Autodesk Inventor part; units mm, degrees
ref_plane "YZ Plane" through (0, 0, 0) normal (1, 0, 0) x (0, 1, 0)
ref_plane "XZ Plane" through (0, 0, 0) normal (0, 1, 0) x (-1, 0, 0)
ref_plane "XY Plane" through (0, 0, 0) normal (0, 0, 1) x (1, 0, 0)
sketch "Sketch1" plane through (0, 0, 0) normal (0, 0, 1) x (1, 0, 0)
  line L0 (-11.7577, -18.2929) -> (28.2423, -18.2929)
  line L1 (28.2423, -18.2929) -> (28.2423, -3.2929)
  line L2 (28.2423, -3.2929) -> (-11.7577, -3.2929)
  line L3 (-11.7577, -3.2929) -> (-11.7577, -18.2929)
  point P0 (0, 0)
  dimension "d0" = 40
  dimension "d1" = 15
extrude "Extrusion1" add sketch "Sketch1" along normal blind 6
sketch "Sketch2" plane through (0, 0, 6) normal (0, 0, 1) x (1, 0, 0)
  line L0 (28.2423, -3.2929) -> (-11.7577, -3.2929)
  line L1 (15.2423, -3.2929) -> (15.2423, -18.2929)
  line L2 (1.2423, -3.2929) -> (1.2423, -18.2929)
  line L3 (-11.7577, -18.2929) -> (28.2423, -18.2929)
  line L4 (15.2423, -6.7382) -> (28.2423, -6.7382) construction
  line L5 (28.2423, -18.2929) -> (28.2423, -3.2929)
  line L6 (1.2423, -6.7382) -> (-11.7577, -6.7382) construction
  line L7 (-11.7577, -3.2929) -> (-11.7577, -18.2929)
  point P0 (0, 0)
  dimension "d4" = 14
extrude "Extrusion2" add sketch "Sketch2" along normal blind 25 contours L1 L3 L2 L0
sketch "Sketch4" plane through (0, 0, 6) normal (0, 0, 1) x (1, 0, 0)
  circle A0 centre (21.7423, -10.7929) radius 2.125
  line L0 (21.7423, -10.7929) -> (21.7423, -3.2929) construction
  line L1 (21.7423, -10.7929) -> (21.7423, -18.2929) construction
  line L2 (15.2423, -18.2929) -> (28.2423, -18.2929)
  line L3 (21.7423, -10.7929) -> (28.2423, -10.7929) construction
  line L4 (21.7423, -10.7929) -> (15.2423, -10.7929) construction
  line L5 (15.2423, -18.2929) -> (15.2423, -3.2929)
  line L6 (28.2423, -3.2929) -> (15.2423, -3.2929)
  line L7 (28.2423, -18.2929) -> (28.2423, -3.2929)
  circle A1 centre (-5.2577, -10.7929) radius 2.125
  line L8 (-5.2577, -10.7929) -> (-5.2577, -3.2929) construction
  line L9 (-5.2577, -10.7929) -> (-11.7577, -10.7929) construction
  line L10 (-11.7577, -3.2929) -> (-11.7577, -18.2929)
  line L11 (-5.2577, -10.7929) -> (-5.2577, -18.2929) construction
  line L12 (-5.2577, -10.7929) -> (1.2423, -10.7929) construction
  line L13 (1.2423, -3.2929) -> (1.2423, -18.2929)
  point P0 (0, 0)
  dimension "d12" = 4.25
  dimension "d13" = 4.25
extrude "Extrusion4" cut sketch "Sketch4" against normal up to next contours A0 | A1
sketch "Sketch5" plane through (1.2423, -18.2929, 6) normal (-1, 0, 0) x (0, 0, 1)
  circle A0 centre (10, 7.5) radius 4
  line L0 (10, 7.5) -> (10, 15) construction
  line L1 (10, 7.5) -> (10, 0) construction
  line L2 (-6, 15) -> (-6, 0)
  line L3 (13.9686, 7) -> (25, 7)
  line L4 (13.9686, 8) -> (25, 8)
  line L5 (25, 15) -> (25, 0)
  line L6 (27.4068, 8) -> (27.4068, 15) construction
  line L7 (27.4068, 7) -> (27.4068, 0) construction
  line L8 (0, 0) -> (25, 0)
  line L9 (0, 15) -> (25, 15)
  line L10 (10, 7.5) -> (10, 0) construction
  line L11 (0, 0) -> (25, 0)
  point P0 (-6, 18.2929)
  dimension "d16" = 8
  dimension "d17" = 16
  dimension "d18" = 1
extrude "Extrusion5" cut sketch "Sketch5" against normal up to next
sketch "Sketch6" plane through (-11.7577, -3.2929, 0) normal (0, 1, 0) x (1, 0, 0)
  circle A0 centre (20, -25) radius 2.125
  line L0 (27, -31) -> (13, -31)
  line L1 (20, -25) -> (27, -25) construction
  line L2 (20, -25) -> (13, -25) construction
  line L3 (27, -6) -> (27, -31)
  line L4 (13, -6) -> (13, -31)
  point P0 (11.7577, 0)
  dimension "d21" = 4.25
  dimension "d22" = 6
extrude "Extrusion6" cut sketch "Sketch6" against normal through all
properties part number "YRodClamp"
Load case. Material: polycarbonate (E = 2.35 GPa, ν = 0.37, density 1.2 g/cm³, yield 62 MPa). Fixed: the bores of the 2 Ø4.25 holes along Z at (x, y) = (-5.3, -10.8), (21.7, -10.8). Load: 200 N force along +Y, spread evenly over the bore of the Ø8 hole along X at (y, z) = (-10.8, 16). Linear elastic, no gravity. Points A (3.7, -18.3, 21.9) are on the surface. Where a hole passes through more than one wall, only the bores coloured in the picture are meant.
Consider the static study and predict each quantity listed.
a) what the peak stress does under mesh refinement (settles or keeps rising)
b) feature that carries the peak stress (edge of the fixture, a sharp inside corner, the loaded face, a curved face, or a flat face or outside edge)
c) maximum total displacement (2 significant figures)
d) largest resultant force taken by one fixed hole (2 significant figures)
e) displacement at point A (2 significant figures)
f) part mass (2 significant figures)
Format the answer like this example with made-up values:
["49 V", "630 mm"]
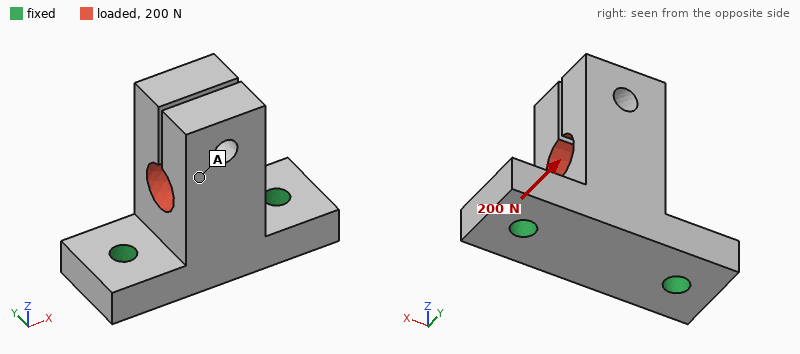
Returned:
["keeps rising", "edge of the fixture", "0.54 mm", "100 N", "0.35 mm", "9.1 g"]
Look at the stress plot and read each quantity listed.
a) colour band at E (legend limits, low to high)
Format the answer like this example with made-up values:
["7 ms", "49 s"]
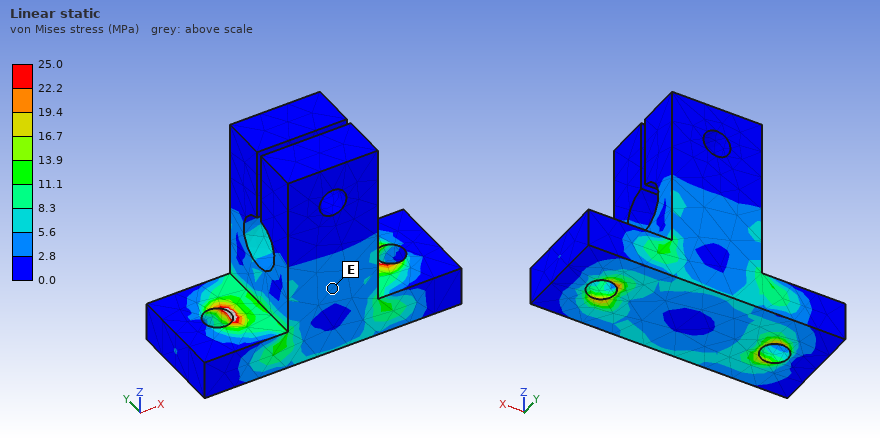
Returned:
["2.8 to 5.6 MPa"]
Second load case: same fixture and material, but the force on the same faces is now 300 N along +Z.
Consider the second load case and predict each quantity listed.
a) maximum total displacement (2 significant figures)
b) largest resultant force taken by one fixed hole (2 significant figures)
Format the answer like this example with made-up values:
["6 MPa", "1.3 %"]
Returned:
["0.19 mm", "160 N"]
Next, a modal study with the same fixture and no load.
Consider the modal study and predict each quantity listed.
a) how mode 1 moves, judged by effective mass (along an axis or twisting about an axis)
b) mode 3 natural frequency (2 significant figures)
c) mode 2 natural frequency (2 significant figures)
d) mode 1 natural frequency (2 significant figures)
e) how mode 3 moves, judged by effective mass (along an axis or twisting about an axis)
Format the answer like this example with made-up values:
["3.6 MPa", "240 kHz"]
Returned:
["along Y", "2700 Hz", "1700 Hz", "1300 Hz", "along X"]
